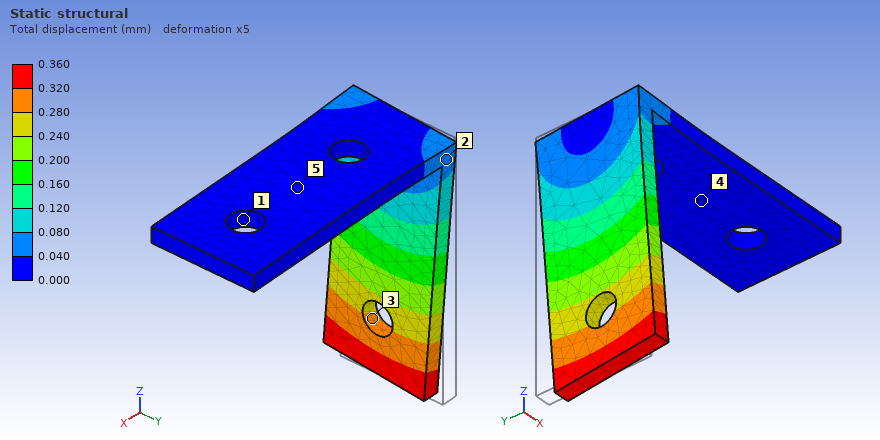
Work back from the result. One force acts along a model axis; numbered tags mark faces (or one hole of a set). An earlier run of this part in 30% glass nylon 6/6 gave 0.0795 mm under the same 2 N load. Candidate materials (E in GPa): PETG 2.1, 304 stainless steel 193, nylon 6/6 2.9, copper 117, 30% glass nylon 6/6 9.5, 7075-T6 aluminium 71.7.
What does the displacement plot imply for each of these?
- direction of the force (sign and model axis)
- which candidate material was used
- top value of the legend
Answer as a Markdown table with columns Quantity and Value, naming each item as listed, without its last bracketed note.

| Quantity | Value |
|---|---|
| direction of the force | -Y |
| which candidate material was used | PETG |
| top value of the legend | 0.360 mm |
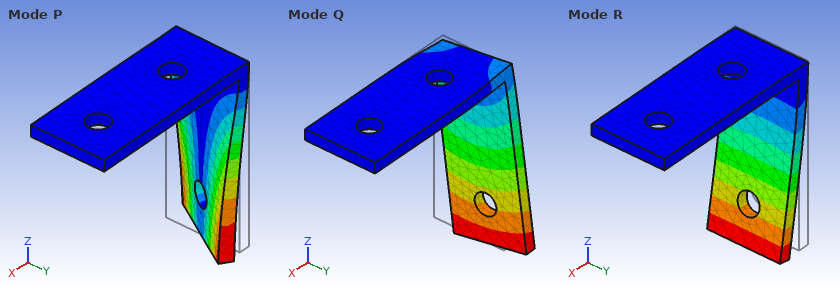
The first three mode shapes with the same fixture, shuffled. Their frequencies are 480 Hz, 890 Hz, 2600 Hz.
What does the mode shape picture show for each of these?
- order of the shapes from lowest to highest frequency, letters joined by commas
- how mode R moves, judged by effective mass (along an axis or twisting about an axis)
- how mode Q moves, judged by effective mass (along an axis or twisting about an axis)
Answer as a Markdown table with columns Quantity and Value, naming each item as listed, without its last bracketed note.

| Quantity | Value |
|---|---|
| order of the shapes from lowest to highest frequency, letters joined by commas | R, Q, P |
| how mode R moves, judged by effective mass | along X |
| how mode Q moves, judged by effective mass | along Y |
